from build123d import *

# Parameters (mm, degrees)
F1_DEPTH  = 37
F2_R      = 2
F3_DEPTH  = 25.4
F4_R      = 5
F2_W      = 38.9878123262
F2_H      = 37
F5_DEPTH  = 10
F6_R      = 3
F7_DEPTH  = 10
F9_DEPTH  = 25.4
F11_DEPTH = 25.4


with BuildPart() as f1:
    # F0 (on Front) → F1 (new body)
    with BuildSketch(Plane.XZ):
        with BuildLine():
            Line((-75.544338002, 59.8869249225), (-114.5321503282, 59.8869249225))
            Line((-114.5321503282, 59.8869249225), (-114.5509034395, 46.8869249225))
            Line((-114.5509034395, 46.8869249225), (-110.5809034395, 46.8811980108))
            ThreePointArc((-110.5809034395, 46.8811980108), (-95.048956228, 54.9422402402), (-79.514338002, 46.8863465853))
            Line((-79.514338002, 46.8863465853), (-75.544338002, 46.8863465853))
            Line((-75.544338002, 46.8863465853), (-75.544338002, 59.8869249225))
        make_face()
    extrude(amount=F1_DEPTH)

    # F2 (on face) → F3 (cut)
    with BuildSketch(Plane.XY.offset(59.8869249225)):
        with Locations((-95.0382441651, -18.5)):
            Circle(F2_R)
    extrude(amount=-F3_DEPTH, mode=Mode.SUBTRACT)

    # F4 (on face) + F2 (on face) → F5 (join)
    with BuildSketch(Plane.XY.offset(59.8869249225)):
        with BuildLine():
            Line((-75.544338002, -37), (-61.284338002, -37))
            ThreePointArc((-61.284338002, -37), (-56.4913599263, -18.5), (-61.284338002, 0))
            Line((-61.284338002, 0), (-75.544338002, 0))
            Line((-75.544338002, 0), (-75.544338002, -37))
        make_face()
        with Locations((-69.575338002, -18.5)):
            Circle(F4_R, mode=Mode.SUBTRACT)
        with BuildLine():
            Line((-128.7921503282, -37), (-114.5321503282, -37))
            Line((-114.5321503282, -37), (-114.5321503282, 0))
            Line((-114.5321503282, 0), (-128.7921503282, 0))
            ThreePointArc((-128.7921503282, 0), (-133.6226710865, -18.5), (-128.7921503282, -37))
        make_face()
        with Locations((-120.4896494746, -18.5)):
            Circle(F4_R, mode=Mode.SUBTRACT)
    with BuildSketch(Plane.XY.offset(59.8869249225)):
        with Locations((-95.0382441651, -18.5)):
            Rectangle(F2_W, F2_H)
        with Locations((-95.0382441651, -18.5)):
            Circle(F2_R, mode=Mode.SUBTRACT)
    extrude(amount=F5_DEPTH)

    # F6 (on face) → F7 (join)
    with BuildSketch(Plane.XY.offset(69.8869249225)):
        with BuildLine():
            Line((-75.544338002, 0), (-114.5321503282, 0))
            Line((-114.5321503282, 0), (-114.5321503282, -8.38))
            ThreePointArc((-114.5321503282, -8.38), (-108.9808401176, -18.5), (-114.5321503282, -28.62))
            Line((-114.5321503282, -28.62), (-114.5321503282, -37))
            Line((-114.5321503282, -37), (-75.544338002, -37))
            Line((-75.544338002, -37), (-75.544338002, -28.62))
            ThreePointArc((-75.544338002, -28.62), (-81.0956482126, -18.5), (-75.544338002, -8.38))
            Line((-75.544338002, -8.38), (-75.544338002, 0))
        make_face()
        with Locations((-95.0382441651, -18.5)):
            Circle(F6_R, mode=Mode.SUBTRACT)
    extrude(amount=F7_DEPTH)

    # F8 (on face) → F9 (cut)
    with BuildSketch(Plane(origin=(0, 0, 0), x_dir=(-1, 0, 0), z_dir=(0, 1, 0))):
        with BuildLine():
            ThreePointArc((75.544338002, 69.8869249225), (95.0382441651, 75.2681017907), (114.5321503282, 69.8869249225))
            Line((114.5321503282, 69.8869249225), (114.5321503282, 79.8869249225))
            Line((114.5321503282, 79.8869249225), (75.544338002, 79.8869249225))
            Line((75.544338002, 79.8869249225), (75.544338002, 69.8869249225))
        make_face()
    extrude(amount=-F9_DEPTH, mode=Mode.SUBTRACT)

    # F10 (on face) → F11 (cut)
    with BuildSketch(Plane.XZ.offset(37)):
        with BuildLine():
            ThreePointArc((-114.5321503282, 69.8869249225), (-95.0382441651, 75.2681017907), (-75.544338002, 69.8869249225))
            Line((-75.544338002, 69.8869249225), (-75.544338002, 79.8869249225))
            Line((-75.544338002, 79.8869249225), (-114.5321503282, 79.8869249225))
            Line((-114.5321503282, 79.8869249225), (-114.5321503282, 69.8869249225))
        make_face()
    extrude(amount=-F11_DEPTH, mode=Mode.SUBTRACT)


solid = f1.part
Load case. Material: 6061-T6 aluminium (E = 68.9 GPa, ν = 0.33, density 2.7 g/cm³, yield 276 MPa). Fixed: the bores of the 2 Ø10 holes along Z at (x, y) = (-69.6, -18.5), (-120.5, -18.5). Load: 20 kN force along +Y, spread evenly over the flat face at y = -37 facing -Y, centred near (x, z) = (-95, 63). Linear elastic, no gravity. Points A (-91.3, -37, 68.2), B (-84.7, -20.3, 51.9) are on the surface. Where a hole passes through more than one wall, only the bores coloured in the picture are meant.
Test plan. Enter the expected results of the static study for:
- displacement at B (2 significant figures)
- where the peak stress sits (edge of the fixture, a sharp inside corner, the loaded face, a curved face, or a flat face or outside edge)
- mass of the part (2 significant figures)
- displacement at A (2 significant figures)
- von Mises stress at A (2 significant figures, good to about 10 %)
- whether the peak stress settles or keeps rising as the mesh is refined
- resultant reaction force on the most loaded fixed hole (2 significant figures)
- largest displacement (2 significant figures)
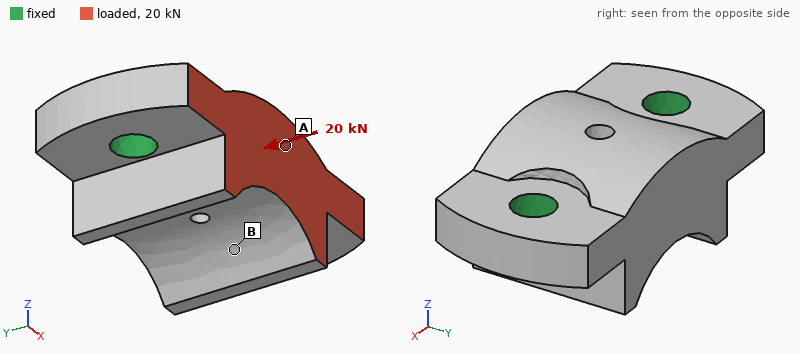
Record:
16 µm
edge of the fixture
120 g
15 µm
24 MPa
keeps rising
10 kN
24 µm
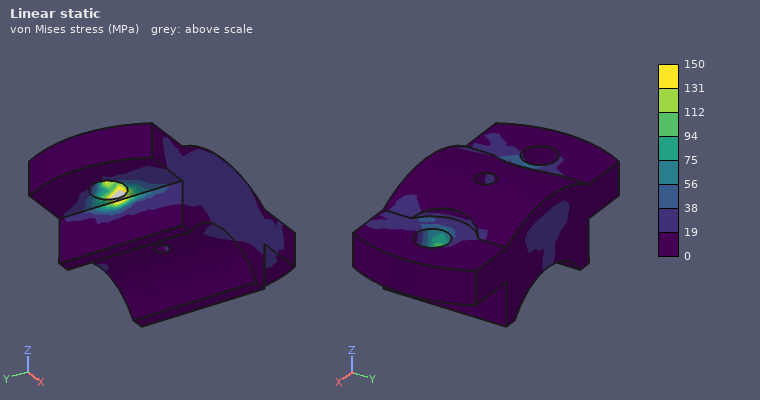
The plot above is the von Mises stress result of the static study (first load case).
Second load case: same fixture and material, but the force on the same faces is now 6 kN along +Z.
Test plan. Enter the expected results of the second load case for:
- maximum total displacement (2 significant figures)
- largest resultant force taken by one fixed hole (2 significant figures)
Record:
38 µm
3.0 kN
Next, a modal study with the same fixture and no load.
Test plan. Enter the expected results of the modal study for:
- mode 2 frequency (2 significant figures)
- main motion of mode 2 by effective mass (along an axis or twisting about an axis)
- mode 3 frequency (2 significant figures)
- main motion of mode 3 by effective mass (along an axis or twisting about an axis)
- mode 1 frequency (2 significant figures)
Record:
16 kHz
along Z
20 kHz
along Y
12 kHz
